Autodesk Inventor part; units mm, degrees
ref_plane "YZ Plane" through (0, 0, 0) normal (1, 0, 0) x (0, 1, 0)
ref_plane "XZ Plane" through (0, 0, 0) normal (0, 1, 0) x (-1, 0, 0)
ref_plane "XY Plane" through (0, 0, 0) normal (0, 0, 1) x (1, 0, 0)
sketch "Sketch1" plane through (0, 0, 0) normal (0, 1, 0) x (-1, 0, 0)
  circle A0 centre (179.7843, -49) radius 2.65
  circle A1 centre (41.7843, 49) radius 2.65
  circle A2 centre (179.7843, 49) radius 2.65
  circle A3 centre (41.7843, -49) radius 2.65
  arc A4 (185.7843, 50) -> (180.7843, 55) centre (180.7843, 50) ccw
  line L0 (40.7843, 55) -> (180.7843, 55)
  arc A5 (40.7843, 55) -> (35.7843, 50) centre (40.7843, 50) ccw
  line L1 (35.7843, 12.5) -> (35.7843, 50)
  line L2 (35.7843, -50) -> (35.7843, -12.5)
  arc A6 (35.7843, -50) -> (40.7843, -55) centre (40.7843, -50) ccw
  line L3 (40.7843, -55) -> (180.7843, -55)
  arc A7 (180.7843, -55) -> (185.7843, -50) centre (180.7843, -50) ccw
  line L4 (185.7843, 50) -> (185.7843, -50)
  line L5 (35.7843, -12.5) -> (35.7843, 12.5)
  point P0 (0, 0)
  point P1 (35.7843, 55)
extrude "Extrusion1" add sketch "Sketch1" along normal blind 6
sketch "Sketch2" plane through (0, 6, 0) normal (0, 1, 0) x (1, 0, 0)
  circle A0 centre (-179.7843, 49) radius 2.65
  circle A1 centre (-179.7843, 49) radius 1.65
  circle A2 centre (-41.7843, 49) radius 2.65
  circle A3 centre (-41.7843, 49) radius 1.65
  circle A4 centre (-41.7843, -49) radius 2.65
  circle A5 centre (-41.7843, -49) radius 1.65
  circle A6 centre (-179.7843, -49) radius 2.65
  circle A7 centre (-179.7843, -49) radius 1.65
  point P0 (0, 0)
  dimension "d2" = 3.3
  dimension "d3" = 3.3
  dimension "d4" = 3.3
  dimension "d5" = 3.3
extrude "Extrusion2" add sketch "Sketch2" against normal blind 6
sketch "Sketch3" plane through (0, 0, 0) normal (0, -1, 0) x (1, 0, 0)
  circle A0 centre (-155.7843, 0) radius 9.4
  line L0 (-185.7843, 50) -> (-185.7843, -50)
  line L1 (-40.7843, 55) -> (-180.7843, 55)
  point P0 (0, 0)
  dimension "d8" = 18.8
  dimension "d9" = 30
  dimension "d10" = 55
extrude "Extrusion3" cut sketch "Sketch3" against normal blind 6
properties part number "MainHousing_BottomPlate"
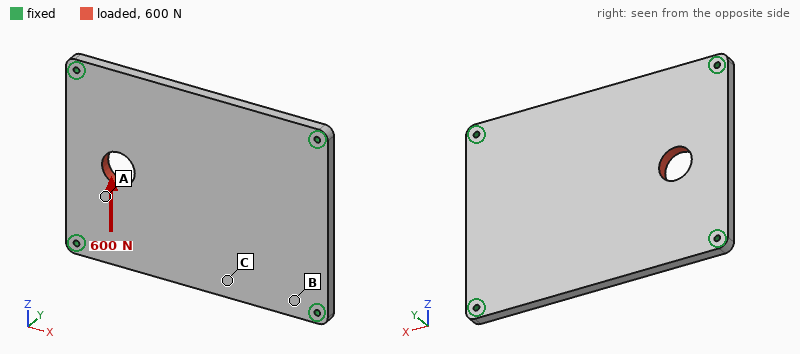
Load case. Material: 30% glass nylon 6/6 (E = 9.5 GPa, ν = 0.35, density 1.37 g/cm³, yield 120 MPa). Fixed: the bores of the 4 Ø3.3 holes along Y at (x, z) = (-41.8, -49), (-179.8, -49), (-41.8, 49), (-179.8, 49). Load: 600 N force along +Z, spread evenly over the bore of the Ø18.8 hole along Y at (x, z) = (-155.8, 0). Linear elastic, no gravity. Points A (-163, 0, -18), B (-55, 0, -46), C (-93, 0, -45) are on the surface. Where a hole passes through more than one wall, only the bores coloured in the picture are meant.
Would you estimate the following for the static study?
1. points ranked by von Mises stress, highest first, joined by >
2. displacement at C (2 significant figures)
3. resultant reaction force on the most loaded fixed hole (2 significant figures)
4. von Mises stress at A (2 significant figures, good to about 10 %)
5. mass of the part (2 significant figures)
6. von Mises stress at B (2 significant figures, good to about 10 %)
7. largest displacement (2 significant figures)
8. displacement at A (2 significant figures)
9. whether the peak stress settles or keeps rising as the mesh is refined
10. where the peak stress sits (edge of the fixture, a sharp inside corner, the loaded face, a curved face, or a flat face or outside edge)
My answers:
A > B > C
6.0 µm
250 N
1.6 MPa
130 g
0.69 MPa
13 µm
9.2 µm
keeps rising
edge of the fixture
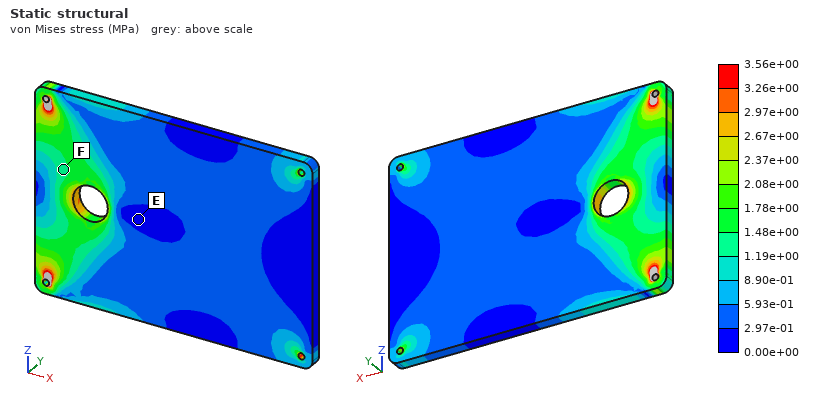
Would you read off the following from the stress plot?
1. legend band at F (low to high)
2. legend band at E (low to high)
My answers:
1.19e+00 to 1.48e+00 MPa
0.00e+00 to 2.97e-01 MPa
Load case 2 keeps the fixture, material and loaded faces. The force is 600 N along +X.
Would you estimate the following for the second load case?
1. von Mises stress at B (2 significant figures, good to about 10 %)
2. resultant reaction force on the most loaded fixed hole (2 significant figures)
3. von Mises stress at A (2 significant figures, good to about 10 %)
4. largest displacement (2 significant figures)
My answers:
1.1 MPa
190 N
1.2 MPa
16 µm
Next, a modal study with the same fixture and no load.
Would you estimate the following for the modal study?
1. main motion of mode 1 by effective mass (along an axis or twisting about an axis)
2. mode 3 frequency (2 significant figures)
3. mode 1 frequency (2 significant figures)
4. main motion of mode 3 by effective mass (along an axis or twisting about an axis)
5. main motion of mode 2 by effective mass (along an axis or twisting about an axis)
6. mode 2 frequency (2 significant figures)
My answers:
along Y
1400 Hz
600 Hz
twisting about Z
twisting about X
1000 Hz
